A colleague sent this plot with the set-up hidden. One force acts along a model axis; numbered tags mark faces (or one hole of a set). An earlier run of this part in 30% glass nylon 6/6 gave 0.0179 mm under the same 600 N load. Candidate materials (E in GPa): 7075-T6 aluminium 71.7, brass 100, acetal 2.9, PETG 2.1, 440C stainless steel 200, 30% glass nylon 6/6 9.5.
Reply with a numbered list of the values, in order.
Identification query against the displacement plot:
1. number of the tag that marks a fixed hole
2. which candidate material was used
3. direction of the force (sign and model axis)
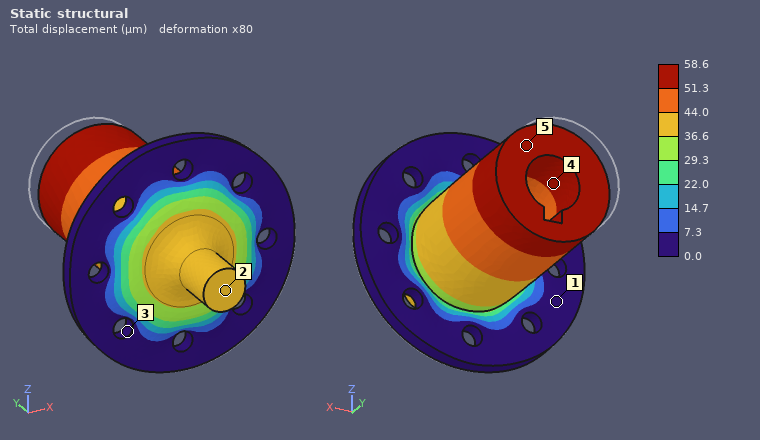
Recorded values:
1. 3
2. acetal
3. -Y
